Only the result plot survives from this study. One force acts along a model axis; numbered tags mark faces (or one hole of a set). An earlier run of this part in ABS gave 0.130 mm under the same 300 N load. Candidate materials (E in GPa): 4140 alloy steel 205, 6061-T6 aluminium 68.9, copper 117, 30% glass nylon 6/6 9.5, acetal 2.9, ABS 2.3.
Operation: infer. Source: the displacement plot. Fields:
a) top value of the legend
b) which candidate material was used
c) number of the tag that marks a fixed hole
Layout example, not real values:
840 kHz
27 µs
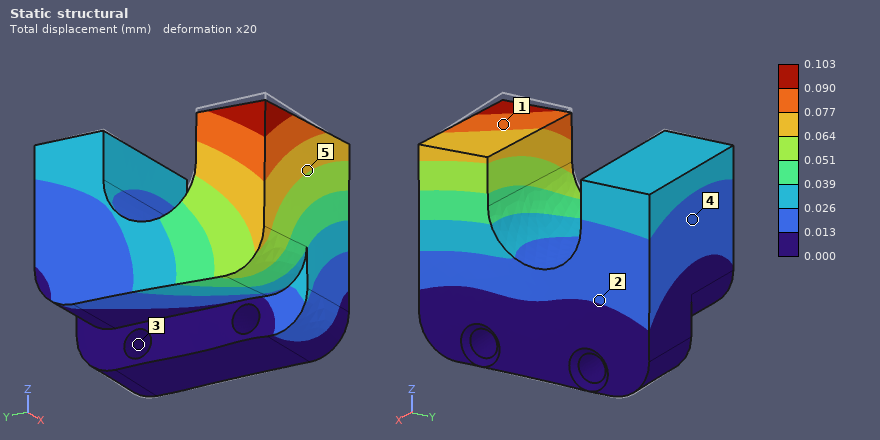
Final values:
0.103 mm
acetal
3
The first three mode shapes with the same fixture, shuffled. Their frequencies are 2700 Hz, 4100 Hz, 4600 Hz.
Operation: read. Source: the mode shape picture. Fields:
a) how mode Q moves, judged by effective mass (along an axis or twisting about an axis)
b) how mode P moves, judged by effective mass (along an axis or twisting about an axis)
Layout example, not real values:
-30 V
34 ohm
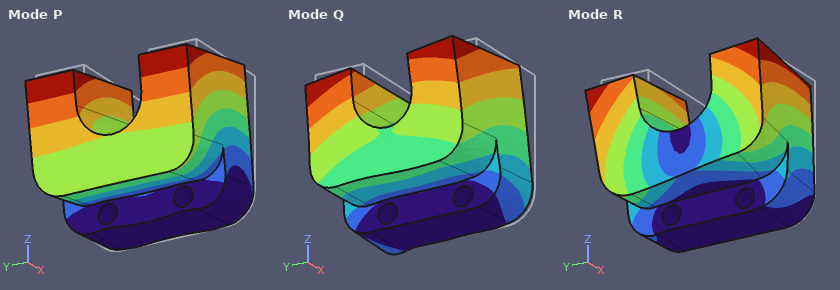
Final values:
along Y
along X
